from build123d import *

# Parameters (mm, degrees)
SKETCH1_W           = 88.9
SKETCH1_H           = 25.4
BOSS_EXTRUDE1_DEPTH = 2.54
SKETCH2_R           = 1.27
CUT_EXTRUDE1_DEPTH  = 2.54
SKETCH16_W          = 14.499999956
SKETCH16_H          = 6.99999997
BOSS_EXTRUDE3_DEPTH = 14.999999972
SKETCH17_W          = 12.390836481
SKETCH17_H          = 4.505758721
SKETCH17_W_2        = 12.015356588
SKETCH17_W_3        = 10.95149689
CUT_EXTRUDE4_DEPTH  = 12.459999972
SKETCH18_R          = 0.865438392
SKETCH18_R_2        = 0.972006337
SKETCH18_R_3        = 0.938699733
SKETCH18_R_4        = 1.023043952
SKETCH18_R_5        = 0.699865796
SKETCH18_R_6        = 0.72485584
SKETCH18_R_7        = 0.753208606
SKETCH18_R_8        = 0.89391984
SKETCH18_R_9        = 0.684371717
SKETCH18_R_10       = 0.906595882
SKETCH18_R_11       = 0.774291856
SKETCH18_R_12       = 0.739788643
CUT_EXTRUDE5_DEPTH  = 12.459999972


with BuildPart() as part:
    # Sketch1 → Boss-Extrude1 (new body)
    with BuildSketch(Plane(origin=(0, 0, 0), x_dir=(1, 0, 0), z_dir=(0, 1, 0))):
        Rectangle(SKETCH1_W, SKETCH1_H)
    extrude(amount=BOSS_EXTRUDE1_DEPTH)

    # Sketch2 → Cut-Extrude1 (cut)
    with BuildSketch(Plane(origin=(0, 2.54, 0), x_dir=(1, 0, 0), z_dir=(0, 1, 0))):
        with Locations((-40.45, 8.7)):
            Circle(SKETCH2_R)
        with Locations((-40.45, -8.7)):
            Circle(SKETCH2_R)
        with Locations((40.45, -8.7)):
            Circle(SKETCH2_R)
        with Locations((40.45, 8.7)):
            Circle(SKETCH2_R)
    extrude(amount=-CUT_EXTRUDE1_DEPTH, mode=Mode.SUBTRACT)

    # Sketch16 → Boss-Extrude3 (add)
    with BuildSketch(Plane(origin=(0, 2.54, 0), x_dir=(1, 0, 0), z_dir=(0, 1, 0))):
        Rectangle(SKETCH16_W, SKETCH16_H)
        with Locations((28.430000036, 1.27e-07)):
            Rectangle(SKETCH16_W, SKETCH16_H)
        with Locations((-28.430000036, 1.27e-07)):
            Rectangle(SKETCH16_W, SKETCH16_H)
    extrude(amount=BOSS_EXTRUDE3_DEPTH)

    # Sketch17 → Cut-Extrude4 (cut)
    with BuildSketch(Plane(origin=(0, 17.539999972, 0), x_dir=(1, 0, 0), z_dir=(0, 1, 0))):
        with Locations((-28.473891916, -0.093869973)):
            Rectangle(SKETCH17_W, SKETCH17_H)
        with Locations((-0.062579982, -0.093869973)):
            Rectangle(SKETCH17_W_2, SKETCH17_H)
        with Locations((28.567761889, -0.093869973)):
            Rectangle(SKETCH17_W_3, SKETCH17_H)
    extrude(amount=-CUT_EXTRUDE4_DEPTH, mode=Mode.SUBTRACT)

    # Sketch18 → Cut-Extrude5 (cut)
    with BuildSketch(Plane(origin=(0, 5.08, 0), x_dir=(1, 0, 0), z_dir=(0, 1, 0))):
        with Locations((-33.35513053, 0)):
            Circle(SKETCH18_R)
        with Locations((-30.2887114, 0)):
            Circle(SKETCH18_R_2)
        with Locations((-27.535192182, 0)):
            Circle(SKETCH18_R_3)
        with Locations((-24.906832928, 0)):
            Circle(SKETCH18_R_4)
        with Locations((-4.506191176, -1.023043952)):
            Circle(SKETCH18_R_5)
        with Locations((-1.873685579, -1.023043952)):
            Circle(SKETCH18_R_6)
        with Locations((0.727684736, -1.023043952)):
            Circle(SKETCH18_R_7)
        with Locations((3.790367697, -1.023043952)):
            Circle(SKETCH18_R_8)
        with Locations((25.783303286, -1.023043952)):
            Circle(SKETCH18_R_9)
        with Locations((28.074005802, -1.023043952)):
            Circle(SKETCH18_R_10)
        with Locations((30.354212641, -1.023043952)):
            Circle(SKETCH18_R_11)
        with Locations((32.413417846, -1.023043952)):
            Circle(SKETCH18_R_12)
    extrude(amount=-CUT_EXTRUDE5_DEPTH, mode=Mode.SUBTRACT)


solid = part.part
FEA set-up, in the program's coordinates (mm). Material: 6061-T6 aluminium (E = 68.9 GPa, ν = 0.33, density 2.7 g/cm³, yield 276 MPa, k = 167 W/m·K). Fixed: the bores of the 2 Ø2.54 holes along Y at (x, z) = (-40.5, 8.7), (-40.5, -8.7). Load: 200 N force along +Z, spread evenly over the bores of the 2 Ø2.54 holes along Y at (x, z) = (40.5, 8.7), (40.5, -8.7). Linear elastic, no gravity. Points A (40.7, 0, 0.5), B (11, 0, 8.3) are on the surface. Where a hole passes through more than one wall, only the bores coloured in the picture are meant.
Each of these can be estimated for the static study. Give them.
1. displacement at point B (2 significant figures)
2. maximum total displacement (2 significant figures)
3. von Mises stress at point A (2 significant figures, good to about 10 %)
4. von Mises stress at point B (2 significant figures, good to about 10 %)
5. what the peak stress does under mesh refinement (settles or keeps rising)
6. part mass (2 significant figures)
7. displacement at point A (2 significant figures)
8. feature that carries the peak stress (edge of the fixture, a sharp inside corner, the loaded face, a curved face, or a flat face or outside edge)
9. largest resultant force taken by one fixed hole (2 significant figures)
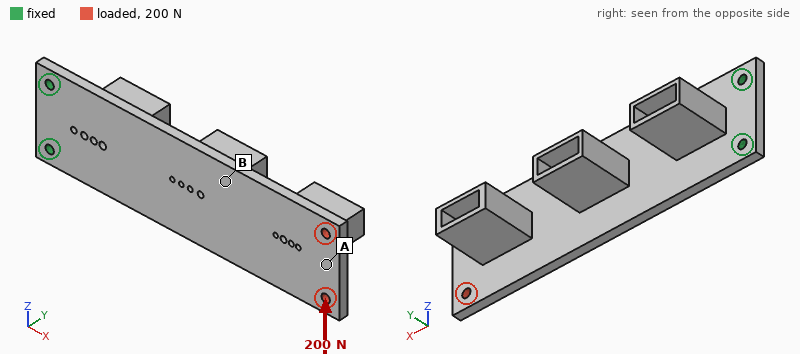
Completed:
0.084 mm
0.18 mm
4.8 MPa
15 MPa
keeps rising
22 g
0.16 mm
edge of the fixture
890 N
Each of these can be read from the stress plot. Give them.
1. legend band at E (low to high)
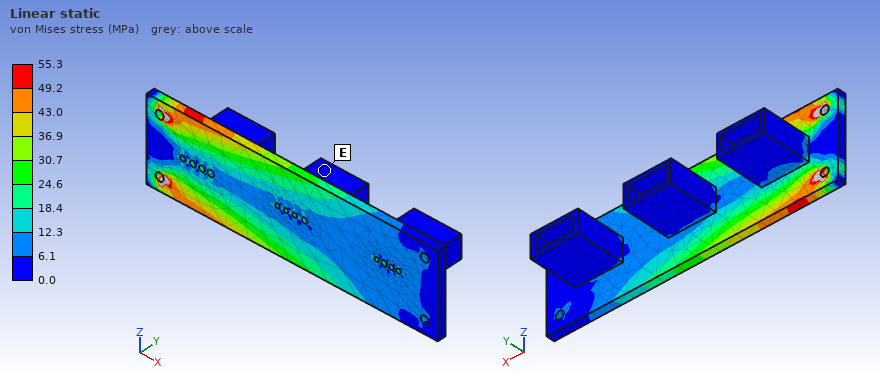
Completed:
0.0 to 6.1 MPa
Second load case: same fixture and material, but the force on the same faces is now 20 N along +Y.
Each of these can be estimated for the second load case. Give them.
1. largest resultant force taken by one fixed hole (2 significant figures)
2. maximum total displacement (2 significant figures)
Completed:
14 N
1.1 mm
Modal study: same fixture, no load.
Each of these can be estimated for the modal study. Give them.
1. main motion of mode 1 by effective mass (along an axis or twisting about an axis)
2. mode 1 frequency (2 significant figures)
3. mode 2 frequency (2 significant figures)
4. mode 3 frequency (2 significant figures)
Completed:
along Y
290 Hz
1700 Hz
1700 Hz
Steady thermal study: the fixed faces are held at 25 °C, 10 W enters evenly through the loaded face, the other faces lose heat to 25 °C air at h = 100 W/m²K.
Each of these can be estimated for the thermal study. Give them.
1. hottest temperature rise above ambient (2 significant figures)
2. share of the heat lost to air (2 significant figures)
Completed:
30 K
82 %
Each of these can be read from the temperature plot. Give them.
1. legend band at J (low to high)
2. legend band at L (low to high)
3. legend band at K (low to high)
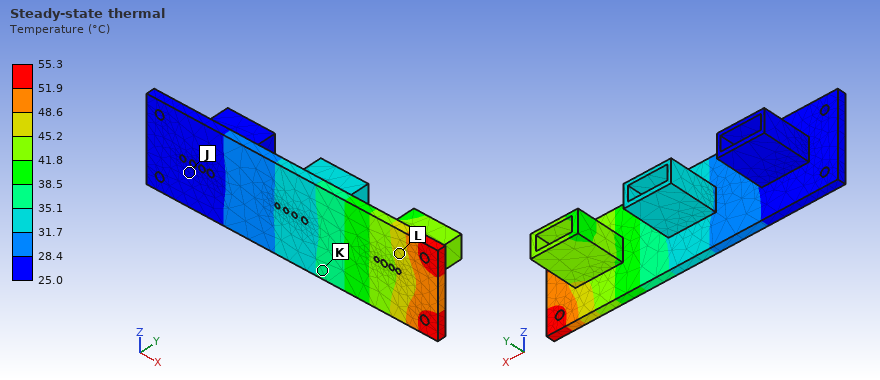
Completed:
25.0 to 28.4 °C
45.2 to 48.6 °C
35.1 to 38.5 °C
